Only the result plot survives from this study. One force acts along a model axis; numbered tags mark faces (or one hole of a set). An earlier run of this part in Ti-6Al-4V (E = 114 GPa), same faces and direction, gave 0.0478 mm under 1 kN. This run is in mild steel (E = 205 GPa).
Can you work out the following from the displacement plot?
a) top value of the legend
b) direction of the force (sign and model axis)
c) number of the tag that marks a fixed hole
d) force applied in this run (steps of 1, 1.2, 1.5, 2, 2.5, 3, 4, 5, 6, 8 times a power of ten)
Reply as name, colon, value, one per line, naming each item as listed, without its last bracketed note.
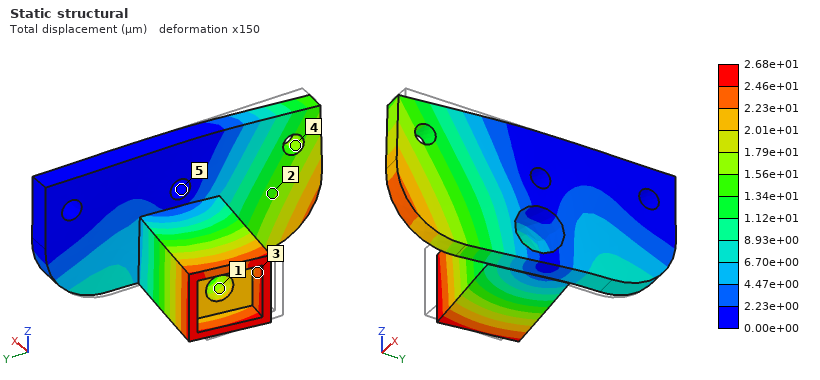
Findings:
top value of the legend: 2.68e+01 µm
direction of the force: +Y
number of the tag that marks a fixed hole: 5
force applied in this run: 1 kN
